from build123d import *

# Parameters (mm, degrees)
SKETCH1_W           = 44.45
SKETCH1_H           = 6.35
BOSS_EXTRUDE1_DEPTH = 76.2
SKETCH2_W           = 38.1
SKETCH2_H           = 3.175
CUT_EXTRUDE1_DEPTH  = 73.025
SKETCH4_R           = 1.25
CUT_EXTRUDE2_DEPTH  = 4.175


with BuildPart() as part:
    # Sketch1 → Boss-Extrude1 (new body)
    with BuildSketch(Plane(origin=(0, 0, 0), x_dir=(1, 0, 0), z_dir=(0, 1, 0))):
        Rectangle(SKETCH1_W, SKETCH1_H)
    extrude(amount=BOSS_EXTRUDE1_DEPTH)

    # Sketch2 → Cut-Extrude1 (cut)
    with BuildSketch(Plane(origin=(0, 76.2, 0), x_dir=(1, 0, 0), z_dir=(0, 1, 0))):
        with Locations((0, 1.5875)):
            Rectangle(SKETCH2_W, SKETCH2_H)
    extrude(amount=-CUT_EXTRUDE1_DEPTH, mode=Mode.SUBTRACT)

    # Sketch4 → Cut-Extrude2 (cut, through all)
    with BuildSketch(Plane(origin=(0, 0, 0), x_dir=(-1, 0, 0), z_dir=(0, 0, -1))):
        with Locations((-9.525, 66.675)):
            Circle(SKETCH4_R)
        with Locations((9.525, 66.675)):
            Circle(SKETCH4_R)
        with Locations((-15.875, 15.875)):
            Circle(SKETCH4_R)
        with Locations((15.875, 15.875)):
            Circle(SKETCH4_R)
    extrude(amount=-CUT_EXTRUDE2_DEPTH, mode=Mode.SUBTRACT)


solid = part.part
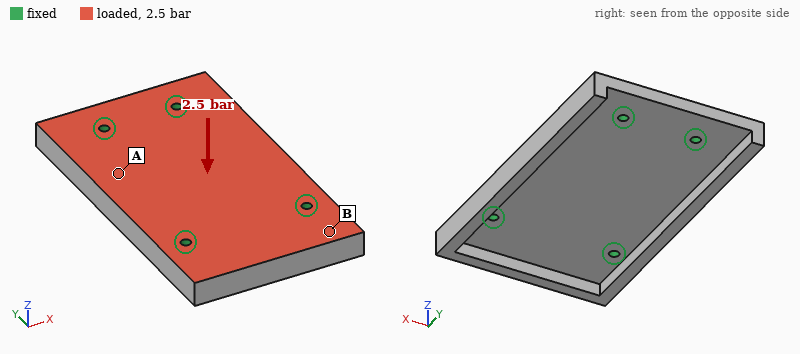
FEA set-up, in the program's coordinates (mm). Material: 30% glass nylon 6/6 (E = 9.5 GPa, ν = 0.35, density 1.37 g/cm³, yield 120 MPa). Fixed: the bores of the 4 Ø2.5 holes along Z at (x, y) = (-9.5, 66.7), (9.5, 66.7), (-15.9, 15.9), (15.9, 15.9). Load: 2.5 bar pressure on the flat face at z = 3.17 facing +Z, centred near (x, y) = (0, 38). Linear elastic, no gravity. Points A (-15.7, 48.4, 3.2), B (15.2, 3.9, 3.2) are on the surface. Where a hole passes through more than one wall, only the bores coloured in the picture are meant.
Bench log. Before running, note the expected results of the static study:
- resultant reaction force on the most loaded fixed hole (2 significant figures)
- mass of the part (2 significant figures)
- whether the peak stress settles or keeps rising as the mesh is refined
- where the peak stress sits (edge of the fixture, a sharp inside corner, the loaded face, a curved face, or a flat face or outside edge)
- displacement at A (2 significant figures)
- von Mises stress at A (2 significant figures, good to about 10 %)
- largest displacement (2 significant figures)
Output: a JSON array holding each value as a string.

["240 N", "17 g", "keeps rising", "edge of the fixture", "0.12 mm", "9.6 MPa", "0.15 mm"]
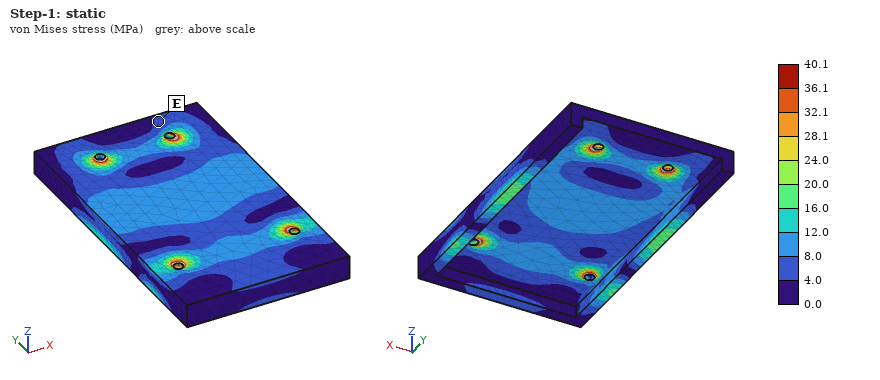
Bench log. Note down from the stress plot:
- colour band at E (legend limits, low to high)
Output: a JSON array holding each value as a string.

["4.0 to 8.0 MPa"]
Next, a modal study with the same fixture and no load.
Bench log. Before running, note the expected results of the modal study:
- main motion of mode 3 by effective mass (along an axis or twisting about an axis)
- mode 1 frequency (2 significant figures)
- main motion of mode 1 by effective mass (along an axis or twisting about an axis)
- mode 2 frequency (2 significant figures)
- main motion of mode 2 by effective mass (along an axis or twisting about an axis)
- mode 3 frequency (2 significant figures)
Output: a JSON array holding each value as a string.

["along Z", "3100 Hz", "along Z", "3700 Hz", "twisting about Y", "4300 Hz"]
